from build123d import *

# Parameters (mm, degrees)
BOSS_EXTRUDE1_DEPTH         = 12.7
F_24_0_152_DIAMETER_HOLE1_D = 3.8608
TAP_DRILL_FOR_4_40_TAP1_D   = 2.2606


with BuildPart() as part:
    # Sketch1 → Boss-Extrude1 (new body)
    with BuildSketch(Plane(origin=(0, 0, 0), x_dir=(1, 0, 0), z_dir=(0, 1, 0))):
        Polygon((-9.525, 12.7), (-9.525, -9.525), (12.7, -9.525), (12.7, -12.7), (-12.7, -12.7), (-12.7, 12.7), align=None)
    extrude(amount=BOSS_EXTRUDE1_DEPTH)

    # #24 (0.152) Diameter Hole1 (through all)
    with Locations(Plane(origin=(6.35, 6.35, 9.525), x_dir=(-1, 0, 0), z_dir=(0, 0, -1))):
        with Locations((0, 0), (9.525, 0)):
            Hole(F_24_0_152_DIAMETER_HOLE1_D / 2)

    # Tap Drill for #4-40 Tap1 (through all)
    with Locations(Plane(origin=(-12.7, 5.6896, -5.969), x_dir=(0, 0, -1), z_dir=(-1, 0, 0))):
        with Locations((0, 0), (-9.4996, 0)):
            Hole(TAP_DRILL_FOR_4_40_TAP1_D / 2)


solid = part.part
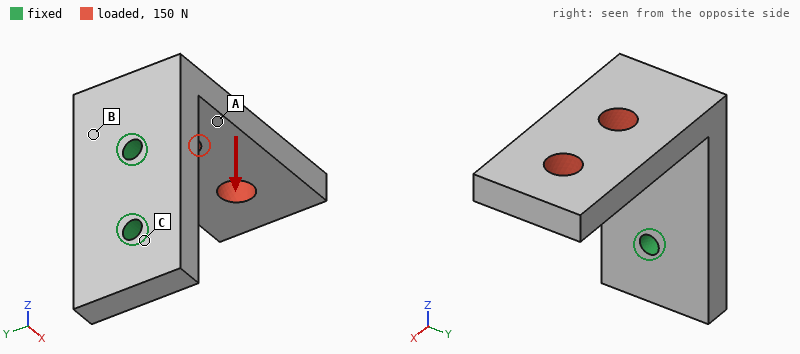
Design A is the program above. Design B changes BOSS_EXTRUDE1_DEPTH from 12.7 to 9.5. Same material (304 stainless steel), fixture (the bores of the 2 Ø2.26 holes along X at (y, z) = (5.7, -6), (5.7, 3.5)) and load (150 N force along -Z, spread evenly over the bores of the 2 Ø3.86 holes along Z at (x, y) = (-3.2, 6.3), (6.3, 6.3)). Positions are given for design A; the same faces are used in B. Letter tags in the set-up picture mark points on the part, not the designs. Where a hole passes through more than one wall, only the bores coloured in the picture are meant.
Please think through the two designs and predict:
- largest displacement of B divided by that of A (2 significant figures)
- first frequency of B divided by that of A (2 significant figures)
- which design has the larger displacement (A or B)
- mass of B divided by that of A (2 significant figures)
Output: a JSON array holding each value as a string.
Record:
["1.4", "1.0", "B", "0.73"]
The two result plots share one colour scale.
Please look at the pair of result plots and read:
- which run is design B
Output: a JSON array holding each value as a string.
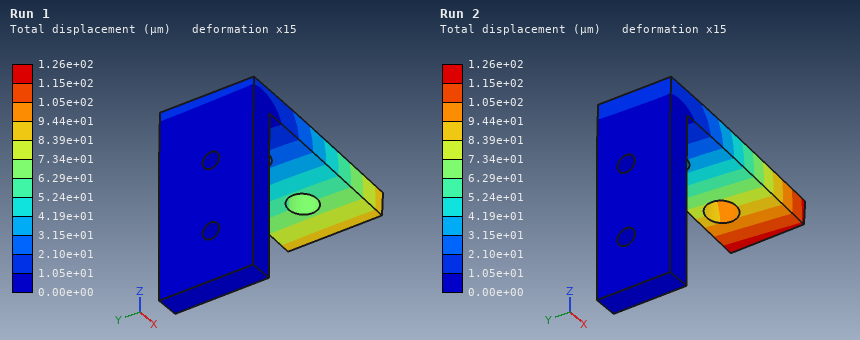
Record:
["Run 2"]
